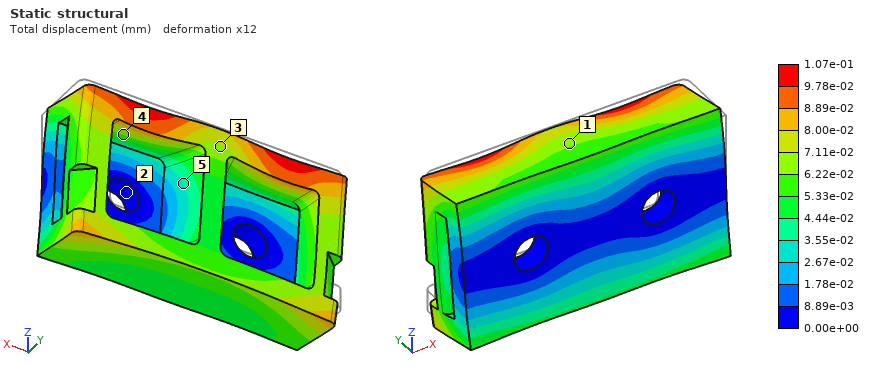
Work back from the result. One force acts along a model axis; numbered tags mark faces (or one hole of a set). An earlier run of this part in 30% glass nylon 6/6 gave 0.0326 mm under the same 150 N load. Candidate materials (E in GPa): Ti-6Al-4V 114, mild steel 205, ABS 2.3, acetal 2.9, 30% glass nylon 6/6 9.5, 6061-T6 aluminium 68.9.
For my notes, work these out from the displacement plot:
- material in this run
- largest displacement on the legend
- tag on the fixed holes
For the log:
acetal
1.07e-01 mm
2
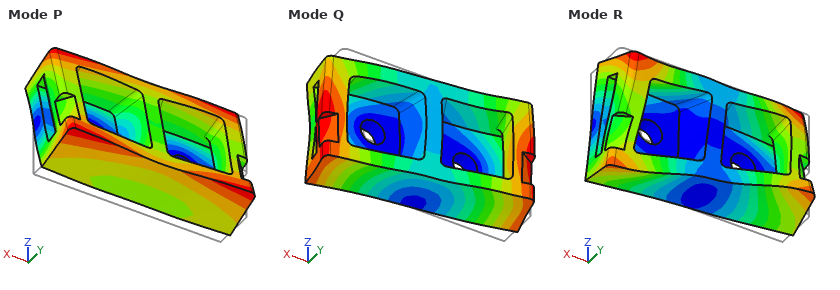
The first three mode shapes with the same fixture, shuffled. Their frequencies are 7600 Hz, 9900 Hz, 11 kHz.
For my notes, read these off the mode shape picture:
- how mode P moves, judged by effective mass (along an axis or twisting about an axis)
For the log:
along Z
